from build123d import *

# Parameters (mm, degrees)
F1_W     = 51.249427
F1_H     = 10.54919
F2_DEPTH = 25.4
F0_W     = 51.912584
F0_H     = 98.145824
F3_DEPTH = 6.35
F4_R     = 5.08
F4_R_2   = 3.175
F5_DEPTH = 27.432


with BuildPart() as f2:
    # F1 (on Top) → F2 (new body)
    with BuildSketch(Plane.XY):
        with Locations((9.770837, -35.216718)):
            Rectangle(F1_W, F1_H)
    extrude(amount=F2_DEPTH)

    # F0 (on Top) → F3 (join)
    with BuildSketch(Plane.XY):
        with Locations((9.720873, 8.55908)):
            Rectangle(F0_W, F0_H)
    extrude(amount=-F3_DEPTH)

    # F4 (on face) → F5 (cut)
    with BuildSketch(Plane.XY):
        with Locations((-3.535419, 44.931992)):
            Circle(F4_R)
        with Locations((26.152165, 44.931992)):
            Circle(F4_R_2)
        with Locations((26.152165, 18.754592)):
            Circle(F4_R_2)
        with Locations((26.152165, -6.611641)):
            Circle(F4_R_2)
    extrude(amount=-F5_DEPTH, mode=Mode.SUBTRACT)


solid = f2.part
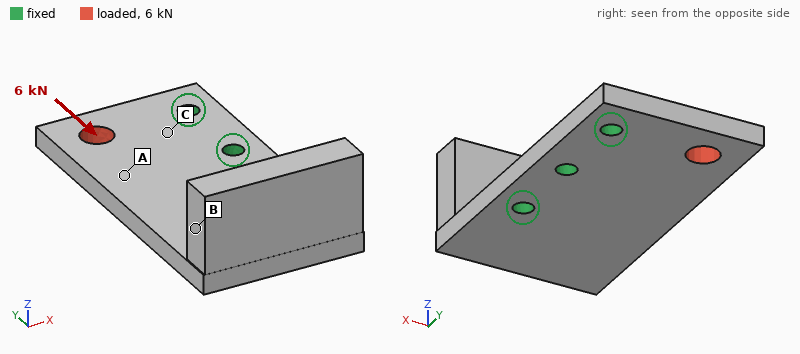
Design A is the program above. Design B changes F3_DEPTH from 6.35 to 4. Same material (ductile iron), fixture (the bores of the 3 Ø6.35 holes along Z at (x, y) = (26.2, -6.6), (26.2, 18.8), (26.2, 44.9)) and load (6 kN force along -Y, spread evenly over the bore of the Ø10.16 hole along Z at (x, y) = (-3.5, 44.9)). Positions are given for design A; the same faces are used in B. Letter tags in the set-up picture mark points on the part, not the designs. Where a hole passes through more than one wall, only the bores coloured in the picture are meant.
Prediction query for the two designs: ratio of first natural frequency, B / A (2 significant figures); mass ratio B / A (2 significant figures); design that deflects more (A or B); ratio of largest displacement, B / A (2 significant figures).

0.55
0.74
B
1.6
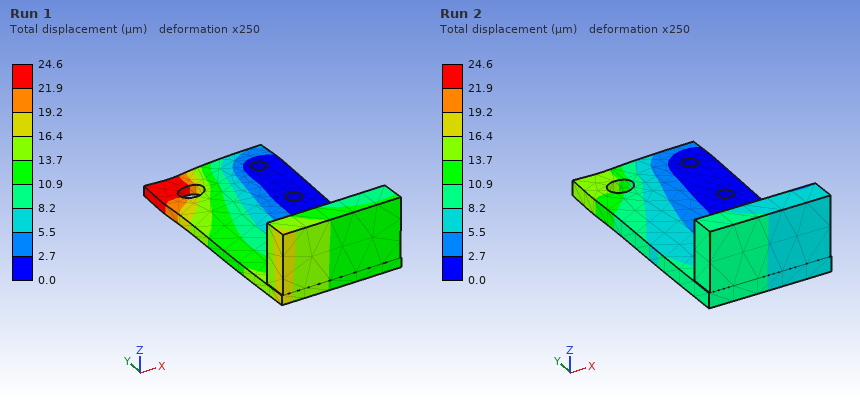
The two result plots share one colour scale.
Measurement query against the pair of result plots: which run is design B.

Run 1
